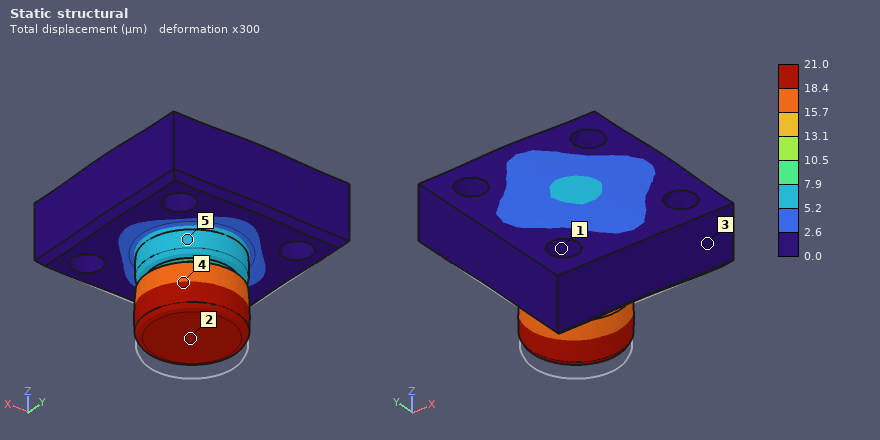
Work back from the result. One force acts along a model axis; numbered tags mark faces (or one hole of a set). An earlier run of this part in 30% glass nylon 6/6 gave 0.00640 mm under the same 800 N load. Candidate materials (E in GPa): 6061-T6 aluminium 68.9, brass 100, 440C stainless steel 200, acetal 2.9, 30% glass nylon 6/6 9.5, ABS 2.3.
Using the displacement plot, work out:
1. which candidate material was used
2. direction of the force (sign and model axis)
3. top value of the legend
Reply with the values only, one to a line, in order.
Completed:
acetal
+Z
21.0 µm
